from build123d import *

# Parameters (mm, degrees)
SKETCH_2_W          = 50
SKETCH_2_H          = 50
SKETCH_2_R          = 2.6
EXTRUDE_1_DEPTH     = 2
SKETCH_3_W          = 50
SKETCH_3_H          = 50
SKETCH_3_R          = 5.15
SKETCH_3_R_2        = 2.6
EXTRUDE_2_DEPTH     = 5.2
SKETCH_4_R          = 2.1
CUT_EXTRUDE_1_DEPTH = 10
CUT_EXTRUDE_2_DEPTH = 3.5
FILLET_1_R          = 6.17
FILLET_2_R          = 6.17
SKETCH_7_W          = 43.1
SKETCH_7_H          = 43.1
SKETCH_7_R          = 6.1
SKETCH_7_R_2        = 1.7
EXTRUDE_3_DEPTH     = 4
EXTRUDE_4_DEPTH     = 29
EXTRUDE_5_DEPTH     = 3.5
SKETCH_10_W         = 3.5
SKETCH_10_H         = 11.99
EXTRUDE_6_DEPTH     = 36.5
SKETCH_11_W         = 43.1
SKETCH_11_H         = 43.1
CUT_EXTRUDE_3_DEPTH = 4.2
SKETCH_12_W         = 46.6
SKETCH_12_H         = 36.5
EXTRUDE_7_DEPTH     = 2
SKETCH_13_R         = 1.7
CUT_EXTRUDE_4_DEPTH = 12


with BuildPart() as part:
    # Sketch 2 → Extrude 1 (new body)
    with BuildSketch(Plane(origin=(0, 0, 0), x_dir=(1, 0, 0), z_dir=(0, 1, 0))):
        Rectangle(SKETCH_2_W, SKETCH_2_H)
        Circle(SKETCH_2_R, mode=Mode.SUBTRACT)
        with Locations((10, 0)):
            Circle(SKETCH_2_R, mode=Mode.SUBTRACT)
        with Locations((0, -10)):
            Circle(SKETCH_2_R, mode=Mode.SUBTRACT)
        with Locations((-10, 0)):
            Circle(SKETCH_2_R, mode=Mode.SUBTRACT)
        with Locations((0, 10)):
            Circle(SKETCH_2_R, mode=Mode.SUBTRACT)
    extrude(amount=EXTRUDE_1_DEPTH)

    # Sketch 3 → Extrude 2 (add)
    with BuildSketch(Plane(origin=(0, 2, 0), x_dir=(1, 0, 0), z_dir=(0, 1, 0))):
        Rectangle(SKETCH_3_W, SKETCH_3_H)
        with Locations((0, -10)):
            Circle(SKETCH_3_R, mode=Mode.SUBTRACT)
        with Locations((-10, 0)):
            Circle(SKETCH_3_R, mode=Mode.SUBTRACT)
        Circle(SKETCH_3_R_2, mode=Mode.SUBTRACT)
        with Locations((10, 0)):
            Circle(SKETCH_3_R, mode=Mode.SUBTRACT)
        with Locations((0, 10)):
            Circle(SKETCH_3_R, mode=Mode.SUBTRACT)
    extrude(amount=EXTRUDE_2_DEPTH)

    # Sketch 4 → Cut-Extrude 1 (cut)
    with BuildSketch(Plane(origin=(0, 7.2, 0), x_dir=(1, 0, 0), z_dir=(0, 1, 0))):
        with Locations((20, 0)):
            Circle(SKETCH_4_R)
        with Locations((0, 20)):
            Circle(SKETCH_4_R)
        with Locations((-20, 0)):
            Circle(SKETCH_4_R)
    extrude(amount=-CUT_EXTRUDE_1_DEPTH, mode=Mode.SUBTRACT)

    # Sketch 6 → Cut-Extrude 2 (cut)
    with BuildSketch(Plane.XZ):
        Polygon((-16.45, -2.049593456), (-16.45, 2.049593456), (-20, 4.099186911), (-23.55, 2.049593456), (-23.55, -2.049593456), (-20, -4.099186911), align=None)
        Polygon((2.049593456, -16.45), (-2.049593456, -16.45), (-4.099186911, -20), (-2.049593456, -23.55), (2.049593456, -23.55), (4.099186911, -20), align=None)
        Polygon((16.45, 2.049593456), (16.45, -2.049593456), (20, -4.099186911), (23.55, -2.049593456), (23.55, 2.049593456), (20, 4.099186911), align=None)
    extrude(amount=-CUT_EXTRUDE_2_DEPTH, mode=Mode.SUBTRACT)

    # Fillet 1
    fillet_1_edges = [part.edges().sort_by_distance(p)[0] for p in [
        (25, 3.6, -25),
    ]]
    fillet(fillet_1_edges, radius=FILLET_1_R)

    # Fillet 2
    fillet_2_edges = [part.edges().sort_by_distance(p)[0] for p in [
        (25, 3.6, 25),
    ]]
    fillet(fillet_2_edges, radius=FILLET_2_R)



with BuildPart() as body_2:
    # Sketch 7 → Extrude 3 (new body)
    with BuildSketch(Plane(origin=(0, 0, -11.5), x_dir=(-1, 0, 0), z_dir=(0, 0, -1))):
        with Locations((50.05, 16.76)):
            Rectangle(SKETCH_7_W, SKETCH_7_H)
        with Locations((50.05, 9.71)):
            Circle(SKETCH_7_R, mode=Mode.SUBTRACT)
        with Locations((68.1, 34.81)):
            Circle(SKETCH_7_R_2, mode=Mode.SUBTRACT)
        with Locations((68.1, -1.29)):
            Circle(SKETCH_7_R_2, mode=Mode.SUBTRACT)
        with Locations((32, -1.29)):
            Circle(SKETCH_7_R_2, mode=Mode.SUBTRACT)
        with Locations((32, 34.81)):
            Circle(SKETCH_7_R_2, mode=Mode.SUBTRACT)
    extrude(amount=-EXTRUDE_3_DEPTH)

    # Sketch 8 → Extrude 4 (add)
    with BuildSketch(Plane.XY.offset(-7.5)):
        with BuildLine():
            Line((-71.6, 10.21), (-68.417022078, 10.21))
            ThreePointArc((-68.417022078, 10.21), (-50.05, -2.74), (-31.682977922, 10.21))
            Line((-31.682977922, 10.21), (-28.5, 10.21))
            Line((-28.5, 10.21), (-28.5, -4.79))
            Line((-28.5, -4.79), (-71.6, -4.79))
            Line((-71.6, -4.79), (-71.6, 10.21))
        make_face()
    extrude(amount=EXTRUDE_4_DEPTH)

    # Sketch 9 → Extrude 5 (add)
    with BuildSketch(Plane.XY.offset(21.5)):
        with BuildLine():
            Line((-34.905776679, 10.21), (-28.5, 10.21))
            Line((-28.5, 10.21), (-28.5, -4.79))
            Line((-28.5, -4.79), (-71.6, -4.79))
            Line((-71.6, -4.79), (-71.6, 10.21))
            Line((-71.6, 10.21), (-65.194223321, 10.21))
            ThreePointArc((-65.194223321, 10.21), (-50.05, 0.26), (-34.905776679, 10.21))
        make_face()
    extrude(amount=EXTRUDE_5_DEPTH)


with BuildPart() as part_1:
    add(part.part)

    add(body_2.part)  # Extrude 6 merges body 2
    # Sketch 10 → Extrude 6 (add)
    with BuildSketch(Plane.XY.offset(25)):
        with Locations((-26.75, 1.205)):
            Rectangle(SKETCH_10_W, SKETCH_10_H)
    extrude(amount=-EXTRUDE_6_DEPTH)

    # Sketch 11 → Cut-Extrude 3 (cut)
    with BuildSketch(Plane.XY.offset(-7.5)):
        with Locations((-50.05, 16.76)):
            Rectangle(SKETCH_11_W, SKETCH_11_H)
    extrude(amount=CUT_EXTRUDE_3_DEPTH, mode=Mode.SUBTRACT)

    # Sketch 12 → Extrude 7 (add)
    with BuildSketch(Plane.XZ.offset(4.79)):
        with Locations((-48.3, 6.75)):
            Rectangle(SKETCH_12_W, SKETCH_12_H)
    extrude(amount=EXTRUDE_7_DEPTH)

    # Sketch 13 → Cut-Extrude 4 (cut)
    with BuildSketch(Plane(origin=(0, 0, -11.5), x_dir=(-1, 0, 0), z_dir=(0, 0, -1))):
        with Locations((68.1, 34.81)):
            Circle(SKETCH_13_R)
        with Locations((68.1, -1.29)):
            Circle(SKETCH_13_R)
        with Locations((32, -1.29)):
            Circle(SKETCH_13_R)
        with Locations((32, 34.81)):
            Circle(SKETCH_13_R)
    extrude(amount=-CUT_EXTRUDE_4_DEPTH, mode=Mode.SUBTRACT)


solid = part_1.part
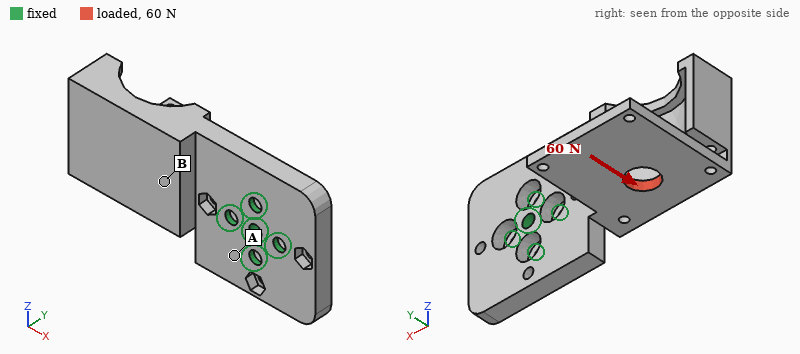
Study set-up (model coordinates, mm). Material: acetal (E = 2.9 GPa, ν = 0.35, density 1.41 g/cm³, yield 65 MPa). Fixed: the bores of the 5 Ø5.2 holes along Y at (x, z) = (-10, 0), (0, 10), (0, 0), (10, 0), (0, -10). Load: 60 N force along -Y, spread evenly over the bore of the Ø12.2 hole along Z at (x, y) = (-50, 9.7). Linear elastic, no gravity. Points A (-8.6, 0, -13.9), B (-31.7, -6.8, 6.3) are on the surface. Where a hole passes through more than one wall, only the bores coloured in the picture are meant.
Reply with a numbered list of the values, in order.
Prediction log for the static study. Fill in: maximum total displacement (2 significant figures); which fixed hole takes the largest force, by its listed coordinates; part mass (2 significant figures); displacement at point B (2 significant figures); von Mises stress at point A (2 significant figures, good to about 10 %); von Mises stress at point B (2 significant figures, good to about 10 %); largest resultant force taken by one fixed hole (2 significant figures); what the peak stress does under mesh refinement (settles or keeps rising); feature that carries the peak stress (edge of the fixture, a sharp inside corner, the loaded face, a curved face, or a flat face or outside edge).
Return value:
1. 1.3 mm
2. (-10, 0)
3. 51 g
4. 0.31 mm
5. 4.0 MPa
6. 2.0 MPa
7. 200 N
8. keeps rising
9. edge of the fixture
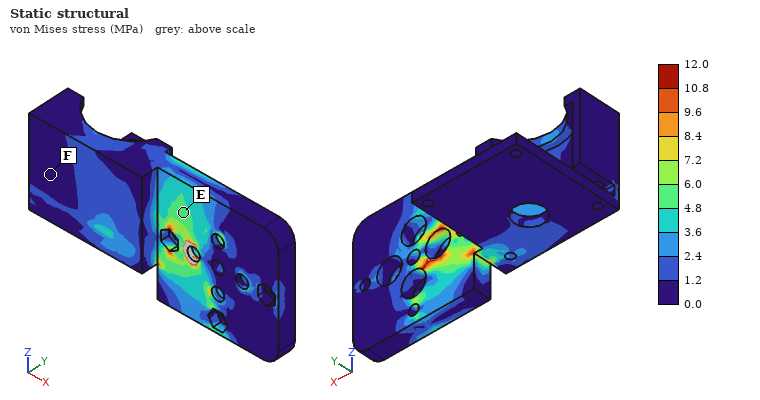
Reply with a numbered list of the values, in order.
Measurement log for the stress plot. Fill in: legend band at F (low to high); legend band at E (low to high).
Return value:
1. 0.0 to 1.2 MPa
2. 4.8 to 6.0 MPa
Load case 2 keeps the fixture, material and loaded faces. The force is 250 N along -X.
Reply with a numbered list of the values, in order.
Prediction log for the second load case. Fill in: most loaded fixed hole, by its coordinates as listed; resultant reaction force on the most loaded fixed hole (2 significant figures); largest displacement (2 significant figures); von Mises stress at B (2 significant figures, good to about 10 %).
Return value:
1. (0, 0)
2. 160 N
3. 1.2 mm
4. 1.8 MPa
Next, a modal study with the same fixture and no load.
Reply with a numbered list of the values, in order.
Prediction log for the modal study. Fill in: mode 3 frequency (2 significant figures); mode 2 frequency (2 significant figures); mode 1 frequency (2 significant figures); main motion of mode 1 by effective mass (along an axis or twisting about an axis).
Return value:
1. 870 Hz
2. 350 Hz
3. 260 Hz
4. along Y
